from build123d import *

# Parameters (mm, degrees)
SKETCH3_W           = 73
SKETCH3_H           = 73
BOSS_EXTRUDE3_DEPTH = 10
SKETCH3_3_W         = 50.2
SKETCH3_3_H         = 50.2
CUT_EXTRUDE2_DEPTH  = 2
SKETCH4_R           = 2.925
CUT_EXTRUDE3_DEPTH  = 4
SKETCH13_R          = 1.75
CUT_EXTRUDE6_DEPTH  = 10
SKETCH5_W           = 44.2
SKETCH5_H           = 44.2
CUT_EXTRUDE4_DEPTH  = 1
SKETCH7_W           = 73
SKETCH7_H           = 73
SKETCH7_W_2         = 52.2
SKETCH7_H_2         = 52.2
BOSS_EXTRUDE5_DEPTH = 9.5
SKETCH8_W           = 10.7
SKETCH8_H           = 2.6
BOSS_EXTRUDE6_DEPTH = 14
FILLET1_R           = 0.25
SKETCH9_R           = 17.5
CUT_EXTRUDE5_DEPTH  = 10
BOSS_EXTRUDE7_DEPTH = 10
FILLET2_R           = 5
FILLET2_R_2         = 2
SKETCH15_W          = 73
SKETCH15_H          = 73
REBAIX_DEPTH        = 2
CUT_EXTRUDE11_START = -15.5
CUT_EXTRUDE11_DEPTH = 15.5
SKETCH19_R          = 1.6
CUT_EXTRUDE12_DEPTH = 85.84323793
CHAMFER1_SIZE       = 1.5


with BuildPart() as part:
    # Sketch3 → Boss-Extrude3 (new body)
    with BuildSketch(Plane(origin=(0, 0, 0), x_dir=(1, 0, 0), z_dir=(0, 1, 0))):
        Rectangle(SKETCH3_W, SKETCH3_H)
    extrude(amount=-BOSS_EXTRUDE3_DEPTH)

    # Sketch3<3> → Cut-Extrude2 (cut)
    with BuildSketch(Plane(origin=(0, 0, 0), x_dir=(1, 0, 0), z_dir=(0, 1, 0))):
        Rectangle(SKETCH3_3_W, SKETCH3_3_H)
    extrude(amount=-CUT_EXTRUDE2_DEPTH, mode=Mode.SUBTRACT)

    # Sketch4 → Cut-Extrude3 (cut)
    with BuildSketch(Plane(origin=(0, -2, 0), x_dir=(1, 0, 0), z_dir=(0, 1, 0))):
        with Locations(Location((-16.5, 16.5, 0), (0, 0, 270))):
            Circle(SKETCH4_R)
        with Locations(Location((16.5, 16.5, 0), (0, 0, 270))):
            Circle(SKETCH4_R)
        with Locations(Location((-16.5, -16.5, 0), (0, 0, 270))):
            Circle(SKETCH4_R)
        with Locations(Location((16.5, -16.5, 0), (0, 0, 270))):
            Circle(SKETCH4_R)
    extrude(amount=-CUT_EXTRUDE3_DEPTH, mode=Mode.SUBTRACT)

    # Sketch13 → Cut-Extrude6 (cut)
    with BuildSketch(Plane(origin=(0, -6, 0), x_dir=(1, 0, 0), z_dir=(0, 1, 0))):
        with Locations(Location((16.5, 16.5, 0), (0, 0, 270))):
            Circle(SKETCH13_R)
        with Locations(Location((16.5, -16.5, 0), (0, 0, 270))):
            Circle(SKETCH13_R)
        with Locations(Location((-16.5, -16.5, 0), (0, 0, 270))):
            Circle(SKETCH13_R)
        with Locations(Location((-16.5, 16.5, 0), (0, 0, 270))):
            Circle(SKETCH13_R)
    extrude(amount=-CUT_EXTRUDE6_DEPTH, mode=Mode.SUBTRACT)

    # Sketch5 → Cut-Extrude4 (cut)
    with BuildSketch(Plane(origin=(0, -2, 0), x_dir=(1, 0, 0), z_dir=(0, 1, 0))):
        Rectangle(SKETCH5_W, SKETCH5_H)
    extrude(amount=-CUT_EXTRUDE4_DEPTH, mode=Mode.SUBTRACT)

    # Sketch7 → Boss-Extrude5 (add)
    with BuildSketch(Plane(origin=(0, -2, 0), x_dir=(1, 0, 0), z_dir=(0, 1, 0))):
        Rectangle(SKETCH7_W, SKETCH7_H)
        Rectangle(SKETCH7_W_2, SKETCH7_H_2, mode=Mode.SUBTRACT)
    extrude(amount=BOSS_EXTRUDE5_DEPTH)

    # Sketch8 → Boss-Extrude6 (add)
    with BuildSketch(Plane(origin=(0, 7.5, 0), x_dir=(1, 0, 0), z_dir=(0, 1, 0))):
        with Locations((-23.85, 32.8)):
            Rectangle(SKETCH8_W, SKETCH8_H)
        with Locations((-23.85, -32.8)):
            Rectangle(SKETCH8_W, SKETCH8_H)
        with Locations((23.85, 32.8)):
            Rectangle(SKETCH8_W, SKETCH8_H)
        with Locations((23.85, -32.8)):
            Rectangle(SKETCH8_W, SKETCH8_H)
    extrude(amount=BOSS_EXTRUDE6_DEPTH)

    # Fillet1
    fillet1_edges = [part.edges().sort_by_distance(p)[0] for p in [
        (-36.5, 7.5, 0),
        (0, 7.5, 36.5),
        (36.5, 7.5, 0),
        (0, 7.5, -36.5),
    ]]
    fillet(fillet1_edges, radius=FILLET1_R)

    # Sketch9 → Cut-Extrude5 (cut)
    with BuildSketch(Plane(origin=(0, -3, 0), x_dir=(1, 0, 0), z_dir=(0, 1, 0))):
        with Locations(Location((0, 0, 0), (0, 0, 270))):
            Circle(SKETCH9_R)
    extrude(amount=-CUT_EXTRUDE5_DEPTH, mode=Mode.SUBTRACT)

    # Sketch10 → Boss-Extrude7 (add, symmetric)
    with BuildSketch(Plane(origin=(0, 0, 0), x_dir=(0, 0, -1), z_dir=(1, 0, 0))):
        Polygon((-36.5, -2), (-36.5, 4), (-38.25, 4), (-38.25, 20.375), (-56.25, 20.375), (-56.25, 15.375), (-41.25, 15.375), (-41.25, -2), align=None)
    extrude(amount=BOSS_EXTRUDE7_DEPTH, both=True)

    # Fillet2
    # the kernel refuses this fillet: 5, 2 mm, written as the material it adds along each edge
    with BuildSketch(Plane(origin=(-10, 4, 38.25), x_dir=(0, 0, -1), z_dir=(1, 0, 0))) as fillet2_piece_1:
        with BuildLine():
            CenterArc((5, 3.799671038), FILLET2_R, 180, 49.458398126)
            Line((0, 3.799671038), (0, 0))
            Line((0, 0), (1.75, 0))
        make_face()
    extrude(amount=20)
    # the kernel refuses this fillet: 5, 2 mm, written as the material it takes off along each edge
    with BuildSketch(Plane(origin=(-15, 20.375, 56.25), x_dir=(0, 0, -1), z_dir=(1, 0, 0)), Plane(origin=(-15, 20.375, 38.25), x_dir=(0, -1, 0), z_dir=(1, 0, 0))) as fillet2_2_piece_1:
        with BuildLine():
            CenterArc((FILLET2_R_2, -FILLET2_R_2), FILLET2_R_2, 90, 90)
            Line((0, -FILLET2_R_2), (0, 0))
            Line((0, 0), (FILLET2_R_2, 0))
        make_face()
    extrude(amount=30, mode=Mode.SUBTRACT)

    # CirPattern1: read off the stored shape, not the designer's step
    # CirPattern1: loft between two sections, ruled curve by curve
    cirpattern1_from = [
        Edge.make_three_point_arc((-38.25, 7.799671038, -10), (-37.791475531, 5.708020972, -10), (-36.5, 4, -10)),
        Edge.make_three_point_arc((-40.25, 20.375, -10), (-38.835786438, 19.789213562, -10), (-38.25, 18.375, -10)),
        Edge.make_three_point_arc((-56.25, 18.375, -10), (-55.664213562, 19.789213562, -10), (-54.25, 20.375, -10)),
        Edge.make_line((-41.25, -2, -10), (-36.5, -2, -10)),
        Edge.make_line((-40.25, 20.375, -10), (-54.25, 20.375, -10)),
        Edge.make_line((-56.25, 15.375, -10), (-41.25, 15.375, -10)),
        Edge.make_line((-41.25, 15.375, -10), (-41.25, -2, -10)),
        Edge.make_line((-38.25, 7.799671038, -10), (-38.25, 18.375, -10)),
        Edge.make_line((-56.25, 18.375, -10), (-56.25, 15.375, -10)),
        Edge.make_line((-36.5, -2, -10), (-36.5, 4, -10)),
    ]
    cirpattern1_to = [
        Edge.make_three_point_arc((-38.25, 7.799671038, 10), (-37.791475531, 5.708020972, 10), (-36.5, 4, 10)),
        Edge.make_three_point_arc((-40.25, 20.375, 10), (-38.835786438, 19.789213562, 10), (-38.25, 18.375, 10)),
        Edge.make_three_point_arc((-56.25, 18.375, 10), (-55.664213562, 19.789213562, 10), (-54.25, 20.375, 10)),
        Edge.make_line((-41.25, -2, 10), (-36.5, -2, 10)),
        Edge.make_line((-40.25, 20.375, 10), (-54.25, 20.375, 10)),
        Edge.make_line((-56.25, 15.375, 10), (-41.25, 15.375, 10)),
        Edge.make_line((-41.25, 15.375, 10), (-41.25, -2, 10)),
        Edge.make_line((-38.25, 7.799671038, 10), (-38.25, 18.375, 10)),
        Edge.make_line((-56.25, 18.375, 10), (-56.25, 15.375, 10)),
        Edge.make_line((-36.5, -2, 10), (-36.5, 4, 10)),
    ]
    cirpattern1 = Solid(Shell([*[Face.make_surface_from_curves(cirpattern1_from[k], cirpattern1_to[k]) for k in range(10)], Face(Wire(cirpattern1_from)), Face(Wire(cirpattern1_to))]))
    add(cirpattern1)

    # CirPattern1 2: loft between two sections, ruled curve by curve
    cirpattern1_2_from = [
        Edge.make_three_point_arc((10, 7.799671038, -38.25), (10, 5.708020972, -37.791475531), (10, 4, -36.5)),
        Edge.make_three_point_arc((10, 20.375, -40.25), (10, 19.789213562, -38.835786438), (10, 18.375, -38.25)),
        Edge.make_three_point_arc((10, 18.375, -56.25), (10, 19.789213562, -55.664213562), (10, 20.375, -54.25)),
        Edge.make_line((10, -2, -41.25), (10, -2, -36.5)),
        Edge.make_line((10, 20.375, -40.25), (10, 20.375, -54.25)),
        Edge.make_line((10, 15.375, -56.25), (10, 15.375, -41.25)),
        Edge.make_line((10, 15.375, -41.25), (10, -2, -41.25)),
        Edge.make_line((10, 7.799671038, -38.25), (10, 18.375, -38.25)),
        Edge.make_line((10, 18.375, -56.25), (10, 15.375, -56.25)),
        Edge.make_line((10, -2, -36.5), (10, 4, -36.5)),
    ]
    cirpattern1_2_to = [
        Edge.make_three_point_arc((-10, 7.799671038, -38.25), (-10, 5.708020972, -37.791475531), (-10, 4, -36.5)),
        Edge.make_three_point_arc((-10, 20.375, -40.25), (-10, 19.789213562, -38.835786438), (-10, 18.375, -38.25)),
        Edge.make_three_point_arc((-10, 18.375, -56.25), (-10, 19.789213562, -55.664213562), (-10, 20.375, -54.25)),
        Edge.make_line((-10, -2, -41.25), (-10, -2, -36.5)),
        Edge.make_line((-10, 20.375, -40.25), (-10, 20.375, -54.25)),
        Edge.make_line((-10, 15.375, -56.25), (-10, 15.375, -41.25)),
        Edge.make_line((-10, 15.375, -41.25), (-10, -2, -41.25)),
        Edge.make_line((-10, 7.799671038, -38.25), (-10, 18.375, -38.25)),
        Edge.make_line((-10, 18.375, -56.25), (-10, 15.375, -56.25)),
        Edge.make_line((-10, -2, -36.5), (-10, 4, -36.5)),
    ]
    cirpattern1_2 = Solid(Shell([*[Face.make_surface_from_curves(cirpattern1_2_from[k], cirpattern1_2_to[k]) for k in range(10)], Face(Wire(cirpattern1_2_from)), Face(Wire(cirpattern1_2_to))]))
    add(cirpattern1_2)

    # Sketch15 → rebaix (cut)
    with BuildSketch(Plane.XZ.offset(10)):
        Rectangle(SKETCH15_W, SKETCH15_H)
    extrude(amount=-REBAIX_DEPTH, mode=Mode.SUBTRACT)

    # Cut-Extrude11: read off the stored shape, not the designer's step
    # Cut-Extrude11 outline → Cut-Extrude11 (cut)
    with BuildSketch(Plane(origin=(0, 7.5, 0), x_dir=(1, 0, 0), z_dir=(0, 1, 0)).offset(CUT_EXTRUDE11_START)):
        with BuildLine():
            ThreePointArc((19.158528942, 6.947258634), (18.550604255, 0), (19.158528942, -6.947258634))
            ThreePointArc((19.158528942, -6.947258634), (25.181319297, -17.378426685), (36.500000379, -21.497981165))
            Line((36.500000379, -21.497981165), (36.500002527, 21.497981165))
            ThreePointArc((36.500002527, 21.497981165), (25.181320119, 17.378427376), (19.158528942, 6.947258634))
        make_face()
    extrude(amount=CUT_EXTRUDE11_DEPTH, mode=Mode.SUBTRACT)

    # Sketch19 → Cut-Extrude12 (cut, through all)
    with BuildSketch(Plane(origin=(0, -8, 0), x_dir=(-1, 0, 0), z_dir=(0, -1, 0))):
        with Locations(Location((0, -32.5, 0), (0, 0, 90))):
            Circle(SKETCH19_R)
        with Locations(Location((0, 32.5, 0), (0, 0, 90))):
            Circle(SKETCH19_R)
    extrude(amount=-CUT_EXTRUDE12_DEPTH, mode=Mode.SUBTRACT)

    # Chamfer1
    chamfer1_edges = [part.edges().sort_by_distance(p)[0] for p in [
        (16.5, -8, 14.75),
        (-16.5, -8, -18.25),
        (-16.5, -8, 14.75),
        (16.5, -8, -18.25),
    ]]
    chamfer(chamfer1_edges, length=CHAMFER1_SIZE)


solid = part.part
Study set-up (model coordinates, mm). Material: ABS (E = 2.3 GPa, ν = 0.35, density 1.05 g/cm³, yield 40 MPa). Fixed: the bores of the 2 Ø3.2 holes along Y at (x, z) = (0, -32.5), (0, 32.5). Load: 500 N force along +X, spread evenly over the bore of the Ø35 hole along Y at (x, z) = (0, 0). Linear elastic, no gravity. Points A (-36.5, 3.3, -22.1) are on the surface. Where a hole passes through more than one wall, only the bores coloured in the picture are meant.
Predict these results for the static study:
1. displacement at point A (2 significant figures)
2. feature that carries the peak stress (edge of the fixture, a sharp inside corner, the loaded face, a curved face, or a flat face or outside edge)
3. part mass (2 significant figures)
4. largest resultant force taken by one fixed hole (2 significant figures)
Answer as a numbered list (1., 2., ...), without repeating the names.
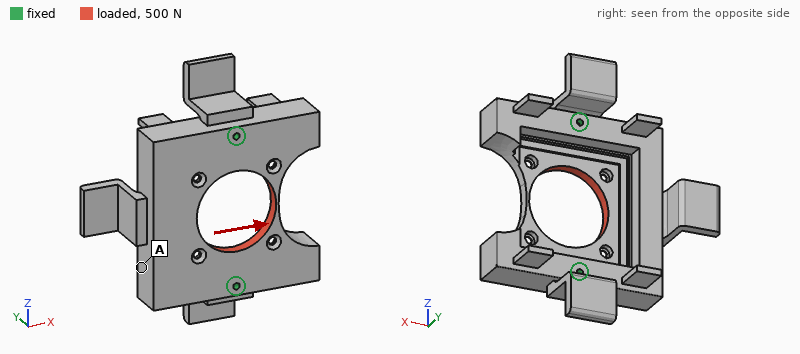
1. 0.052 mm
2. a curved face
3. 55 g
4. 250 N
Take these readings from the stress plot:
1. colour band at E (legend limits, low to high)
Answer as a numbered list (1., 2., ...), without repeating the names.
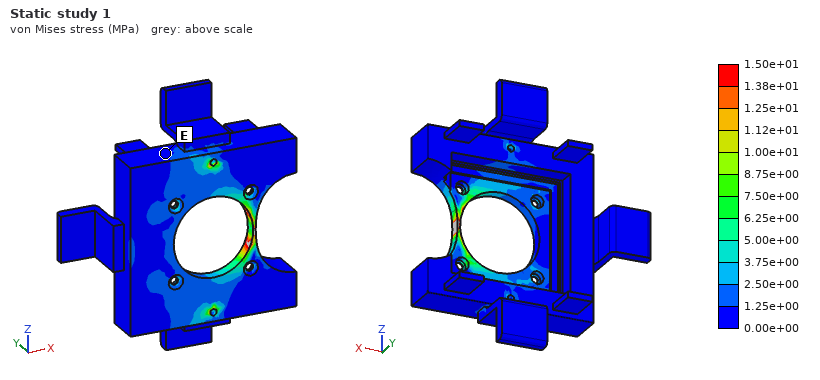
1. 0.00e+00 to 1.25e+00 MPa
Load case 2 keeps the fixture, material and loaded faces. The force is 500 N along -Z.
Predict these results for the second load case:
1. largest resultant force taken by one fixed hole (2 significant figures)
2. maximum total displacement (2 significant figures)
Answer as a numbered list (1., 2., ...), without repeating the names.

1. 250 N
2. 66 µm
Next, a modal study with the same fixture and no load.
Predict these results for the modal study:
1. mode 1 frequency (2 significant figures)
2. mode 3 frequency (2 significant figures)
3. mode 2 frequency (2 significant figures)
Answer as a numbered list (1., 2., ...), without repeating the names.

1. 750 Hz
2. 860 Hz
3. 860 Hz
